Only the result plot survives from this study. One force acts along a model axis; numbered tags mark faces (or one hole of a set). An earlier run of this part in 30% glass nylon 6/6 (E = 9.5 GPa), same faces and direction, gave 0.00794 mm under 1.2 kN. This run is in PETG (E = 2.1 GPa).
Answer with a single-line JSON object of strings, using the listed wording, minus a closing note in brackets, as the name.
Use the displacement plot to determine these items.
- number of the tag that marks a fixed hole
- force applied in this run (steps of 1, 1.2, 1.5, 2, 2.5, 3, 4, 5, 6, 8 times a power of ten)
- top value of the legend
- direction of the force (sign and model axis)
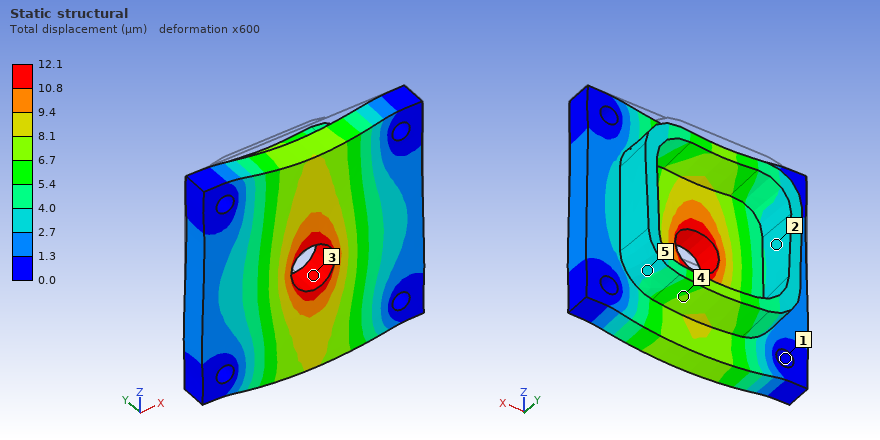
{"number of the tag that marks a fixed hole": "1", "force applied in this run": "400 N", "top value of the legend": "12.1 µm", "direction of the force": "-Z"}
